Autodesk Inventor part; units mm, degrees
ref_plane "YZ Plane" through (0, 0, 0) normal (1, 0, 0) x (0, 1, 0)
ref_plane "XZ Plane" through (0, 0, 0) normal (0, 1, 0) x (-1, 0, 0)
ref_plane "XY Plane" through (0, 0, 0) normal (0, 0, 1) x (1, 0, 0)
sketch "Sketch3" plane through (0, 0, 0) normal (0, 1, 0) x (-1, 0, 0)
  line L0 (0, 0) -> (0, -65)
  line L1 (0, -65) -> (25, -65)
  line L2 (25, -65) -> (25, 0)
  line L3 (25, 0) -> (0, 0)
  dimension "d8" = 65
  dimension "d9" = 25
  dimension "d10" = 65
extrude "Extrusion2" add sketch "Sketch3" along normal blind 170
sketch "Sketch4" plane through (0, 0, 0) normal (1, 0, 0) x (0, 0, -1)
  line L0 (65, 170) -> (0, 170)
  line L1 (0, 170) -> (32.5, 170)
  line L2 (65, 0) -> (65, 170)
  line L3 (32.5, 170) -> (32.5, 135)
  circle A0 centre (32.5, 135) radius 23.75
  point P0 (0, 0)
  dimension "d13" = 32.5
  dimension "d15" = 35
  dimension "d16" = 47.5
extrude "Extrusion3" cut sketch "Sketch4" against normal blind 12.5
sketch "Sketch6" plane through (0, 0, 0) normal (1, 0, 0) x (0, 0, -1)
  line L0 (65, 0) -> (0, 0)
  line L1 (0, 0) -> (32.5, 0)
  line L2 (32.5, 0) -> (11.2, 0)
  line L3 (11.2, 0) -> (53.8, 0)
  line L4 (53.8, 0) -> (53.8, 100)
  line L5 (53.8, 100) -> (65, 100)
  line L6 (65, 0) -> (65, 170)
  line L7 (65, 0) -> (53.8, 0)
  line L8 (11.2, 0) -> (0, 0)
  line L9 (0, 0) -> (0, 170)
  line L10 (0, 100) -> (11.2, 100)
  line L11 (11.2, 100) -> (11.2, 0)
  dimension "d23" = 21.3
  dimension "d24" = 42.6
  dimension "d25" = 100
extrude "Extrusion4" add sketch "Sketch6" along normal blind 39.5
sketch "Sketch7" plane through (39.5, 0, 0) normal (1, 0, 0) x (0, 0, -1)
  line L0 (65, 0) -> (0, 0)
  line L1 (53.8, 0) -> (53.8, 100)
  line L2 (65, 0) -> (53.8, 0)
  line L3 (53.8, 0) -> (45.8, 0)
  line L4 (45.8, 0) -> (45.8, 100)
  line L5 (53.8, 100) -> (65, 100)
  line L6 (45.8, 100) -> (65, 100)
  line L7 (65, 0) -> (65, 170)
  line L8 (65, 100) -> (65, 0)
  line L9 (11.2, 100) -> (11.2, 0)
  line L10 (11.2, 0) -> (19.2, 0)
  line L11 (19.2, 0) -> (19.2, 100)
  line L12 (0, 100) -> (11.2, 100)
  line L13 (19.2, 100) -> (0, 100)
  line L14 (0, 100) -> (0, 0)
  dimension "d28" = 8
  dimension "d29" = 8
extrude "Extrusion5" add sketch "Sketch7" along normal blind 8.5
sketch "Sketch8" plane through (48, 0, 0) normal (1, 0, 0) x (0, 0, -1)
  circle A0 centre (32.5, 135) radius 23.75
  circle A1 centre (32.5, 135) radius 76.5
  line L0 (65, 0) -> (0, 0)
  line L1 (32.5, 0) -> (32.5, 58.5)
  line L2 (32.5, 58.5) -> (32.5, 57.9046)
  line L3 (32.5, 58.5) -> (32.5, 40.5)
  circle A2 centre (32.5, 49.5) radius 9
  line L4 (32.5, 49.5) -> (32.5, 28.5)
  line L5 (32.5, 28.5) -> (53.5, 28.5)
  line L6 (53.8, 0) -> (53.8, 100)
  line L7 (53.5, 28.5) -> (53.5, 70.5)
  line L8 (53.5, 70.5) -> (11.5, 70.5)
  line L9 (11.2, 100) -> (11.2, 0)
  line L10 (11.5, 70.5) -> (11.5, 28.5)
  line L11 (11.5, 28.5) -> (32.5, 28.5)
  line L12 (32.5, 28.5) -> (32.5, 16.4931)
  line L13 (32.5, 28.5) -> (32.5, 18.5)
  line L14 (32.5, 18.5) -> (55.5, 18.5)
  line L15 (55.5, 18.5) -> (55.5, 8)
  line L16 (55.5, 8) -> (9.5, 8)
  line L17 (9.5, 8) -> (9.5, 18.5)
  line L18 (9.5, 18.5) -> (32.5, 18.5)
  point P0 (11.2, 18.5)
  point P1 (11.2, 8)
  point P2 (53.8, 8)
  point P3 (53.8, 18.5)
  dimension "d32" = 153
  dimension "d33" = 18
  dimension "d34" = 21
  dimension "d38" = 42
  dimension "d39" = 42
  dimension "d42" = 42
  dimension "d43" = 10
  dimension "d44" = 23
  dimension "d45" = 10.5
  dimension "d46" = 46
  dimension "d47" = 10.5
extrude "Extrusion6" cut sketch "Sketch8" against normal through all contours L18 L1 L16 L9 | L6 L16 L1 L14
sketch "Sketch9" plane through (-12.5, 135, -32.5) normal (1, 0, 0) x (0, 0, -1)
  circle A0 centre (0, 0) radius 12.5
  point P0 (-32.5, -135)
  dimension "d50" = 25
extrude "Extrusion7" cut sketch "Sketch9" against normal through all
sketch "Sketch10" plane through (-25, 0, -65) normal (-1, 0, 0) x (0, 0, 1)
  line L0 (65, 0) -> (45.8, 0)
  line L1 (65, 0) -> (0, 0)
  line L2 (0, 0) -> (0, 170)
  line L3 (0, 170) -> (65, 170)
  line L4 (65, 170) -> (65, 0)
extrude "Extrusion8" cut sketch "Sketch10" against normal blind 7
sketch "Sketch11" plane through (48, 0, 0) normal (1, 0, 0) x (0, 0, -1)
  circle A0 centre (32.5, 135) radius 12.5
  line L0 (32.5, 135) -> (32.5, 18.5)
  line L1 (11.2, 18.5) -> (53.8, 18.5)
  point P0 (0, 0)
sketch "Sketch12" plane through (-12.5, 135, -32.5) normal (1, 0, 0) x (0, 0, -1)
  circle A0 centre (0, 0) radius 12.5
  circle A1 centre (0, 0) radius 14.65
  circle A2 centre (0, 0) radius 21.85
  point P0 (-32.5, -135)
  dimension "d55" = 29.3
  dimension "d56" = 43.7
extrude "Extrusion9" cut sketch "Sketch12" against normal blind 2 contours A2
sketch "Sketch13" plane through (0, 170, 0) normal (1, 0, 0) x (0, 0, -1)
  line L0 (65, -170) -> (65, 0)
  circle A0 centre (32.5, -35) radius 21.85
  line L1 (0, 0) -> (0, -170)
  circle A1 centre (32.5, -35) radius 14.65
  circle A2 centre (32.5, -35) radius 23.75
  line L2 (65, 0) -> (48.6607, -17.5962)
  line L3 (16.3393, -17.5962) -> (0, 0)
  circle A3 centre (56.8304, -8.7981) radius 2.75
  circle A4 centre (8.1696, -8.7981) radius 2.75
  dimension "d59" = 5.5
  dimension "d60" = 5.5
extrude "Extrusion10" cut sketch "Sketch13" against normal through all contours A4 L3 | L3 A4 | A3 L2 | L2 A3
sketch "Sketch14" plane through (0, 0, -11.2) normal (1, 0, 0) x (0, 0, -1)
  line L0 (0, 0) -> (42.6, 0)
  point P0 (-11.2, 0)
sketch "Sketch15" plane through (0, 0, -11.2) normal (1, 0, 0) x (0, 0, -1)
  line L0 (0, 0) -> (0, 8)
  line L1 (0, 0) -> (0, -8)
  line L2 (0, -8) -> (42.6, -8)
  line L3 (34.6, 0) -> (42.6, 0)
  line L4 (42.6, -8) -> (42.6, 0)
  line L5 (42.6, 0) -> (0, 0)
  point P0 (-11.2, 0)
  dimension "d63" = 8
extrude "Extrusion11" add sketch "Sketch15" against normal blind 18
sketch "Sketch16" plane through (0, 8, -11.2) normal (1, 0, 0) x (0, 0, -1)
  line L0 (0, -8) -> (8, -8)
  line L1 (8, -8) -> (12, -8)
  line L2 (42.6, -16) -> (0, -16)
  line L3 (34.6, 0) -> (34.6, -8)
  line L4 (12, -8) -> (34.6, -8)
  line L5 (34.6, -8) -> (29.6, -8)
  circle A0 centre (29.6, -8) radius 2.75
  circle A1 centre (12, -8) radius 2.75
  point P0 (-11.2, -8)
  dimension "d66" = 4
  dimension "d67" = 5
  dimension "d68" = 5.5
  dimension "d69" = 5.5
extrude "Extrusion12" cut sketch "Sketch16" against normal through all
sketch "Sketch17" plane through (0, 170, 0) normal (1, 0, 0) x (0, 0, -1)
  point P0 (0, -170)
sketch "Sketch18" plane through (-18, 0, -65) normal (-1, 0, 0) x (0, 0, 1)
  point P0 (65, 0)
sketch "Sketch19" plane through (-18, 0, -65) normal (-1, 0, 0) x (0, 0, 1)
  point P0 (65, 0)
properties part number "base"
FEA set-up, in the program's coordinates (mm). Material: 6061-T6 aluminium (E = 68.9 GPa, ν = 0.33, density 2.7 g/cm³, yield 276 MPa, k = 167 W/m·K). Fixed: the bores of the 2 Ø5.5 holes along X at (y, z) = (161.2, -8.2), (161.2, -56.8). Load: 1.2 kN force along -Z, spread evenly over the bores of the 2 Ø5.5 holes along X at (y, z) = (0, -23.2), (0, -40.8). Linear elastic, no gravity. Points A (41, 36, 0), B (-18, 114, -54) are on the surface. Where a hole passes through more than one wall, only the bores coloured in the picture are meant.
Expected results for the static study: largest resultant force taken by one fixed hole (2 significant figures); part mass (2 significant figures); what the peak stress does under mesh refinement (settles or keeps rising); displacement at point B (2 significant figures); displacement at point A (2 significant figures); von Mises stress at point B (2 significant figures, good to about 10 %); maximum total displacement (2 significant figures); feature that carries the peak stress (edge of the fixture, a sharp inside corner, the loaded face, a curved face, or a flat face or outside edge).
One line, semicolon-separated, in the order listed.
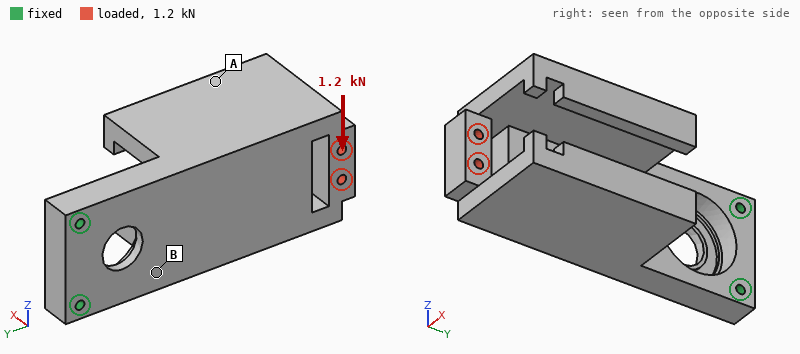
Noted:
3.7 kN; 780 g; keeps rising; 0.024 mm; 0.076 mm; 7.6 MPa; 0.10 mm; edge of the fixture
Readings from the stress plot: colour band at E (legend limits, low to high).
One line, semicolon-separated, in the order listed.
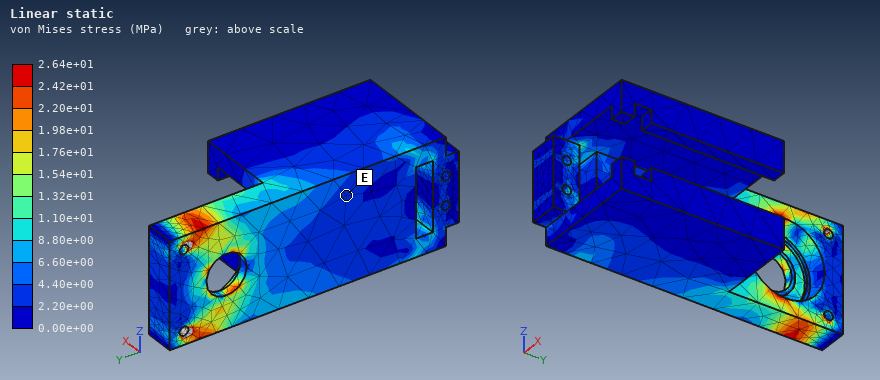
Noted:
2.20e+00 to 4.40e+00 MPa
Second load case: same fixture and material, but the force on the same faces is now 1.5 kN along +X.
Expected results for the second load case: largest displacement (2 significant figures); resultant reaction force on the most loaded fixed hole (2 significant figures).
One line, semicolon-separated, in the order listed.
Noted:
1.8 mm; 980 N
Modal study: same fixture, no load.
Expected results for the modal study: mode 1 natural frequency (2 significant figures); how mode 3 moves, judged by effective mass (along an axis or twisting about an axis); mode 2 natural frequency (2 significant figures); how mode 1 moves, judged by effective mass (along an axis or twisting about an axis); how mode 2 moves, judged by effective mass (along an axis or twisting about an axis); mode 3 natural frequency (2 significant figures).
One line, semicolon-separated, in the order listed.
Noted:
270 Hz; along Z; 710 Hz; along X; along Z; 1300 Hz
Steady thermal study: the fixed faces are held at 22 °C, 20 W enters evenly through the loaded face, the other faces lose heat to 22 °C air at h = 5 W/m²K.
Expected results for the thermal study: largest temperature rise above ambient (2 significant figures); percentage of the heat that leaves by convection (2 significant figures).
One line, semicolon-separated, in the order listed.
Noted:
24 K; 18 %
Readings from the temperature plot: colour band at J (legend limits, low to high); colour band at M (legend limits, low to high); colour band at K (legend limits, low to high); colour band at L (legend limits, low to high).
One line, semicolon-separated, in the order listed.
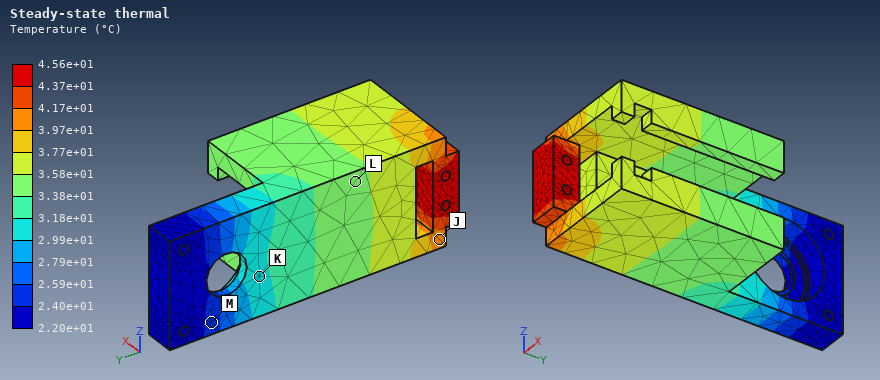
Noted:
3.97e+01 to 4.17e+01 °C; 2.40e+01 to 2.59e+01 °C; 2.99e+01 to 3.18e+01 °C; 3.38e+01 to 3.58e+01 °C
